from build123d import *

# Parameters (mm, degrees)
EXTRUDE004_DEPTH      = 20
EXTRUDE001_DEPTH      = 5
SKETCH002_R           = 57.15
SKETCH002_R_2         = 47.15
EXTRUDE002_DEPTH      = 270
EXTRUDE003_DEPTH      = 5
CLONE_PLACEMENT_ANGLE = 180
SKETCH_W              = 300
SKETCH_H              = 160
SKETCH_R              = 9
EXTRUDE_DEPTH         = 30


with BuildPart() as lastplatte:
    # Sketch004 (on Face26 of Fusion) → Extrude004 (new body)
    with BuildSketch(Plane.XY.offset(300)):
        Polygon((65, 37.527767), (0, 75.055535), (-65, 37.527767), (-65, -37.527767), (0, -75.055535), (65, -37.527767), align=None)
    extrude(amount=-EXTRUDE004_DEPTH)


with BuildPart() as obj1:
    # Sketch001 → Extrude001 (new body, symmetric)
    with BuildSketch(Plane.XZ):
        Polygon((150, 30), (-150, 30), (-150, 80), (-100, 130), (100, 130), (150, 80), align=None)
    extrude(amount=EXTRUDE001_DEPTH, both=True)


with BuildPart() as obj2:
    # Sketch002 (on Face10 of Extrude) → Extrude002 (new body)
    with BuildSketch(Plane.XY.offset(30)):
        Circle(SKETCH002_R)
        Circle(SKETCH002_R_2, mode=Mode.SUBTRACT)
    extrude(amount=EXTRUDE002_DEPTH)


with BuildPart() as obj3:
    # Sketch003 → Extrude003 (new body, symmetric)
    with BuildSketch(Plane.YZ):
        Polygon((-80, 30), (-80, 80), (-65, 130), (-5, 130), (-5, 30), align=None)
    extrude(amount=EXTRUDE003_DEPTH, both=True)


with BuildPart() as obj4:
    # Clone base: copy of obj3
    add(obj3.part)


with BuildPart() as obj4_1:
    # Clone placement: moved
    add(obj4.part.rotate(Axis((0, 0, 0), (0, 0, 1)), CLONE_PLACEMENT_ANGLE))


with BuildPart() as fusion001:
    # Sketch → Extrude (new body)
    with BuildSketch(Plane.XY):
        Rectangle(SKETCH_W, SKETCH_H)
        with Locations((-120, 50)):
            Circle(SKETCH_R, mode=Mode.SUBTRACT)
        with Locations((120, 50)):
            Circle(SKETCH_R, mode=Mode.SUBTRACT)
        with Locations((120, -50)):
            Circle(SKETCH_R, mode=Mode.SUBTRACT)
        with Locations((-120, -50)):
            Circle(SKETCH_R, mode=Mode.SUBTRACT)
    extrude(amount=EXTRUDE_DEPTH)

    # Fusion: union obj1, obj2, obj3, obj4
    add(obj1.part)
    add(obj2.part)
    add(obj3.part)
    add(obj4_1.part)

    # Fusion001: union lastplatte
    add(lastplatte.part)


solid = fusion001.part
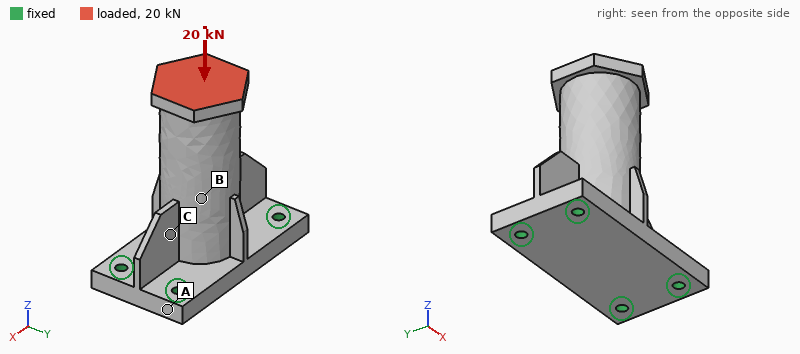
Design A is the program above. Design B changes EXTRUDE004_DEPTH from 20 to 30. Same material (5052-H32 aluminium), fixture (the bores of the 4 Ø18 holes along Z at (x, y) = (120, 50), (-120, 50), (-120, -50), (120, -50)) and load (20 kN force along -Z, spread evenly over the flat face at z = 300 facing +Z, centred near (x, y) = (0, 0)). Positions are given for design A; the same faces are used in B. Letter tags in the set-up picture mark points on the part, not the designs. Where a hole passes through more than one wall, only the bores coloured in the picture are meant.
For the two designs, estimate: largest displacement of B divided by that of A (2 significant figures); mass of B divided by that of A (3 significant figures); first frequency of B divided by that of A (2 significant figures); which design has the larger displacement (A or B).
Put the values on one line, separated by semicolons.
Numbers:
0.90; 1.04; 0.92; A
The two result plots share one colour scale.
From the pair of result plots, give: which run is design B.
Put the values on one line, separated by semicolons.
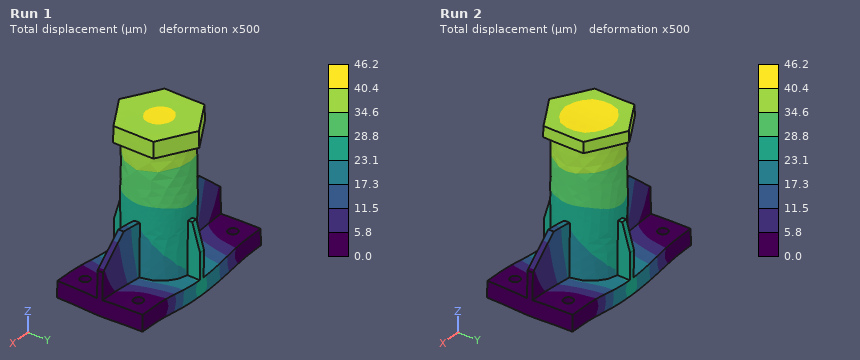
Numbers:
Run 1
